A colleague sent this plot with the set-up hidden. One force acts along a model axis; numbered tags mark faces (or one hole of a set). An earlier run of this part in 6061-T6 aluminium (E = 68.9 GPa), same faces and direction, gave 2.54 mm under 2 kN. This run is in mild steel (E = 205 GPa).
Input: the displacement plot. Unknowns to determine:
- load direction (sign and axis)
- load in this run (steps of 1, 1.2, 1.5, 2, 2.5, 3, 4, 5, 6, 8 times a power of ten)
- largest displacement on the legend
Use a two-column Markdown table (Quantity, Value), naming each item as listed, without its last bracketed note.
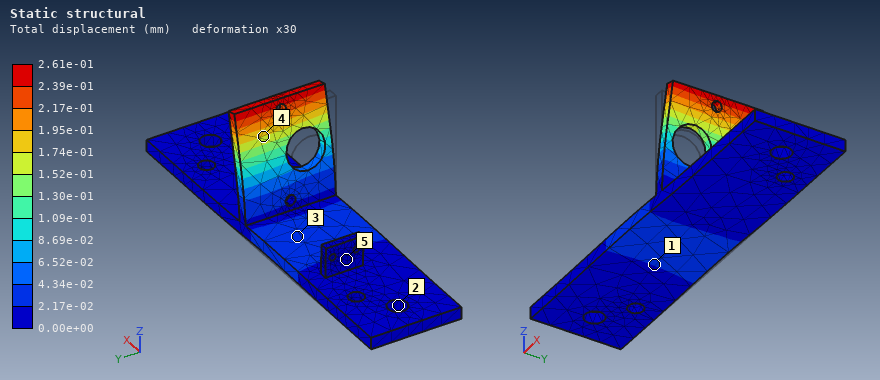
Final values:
| Quantity | Value |
|---|---|
| load direction | +X |
| load in this run | 600 N |
| largest displacement on the legend | 2.61e-01 mm |
